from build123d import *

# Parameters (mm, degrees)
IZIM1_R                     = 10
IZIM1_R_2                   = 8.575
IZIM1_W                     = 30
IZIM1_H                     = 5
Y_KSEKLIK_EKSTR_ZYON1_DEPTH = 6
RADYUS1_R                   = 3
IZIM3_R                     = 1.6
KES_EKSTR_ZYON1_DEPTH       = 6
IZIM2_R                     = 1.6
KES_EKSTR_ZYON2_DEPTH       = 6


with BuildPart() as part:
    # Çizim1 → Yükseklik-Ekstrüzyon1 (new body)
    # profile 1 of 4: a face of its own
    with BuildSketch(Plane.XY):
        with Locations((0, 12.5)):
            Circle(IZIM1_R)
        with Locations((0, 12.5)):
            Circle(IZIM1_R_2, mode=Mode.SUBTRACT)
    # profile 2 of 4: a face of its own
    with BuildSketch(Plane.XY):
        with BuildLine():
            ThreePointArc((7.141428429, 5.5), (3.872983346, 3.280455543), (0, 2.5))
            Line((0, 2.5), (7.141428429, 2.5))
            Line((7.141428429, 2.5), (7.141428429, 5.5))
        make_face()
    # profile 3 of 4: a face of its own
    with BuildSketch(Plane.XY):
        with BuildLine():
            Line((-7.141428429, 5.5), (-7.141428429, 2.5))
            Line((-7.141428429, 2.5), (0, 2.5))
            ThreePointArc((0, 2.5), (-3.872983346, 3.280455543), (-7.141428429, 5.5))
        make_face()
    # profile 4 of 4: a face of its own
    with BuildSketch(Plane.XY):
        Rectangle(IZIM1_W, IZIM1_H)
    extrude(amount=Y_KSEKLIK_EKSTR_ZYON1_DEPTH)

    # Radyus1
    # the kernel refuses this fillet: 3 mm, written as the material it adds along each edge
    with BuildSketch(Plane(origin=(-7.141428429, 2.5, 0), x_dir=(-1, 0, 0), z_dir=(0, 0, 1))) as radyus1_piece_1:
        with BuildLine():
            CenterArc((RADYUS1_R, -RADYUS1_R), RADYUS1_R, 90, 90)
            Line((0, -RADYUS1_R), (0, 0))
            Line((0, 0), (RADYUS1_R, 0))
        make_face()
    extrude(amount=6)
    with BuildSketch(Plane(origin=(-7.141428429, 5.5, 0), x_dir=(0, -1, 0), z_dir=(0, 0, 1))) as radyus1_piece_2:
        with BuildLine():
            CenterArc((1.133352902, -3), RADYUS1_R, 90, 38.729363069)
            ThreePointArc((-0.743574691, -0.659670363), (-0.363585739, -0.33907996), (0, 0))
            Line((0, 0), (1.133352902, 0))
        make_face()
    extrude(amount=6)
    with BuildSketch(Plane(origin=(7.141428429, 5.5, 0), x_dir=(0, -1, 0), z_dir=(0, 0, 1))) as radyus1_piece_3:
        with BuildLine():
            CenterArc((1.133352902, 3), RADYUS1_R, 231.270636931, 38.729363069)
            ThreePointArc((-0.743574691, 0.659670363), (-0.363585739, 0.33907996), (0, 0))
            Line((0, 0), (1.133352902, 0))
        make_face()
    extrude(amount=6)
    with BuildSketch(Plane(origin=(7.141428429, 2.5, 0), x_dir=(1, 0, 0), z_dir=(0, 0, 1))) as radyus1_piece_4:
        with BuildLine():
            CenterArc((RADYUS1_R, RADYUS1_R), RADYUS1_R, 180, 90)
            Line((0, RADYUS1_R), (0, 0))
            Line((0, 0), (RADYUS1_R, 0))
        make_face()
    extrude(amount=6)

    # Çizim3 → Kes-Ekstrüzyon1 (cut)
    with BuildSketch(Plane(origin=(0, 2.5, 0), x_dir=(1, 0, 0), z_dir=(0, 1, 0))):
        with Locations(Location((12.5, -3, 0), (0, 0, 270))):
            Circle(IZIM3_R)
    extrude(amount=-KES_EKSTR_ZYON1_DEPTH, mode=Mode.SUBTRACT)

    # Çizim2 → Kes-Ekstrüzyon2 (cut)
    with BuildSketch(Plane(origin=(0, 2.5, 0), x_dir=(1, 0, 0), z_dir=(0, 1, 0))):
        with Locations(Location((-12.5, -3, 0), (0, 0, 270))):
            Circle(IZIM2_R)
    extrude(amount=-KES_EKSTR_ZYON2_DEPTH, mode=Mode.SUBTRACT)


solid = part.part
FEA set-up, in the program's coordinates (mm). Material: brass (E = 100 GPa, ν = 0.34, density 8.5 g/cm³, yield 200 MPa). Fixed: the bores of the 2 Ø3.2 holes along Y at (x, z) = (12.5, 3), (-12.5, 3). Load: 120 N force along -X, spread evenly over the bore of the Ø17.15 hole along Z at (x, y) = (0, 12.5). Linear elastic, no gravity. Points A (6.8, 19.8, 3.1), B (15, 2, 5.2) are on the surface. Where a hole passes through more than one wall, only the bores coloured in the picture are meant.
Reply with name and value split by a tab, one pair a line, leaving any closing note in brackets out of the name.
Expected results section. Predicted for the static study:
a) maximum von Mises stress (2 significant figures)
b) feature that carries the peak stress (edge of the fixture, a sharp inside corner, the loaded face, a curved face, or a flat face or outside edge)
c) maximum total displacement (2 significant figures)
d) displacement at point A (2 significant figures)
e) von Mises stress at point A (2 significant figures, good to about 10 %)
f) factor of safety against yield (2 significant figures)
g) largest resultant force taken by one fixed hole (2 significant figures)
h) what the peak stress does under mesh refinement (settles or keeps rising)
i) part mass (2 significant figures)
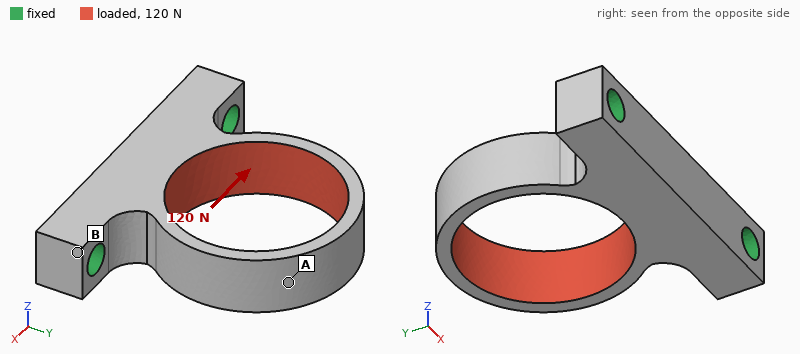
maximum von Mises stress	110 MPa
feature that carries the peak stress	the loaded face
maximum total displacement	76 µm
displacement at point A	74 µm
von Mises stress at point A	45 MPa
factor of safety against yield	1.7
largest resultant force taken by one fixed hole	94 N
what the peak stress does under mesh refinement	settles
part mass	12 g
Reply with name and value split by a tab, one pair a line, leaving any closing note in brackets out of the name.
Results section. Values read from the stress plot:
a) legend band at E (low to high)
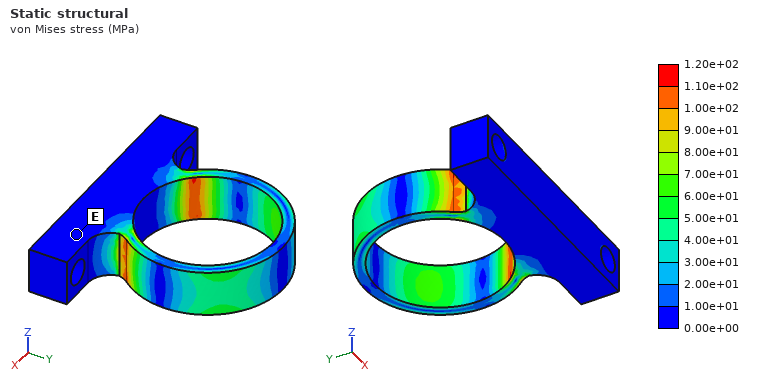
legend band at E	0.00e+00 to 1.00e+01 MPa
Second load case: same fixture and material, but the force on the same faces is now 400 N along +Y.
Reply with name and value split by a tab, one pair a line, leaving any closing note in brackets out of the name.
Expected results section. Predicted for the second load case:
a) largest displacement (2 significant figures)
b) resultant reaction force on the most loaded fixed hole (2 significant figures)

largest displacement	35 µm
resultant reaction force on the most loaded fixed hole	210 N
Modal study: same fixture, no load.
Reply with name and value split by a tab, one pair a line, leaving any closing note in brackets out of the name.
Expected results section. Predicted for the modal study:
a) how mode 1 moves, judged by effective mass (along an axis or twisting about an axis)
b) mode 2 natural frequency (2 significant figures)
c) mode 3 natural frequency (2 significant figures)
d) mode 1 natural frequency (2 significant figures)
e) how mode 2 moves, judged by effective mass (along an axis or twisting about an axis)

how mode 1 moves, judged by effective mass	along X
mode 2 natural frequency	4000 Hz
mode 3 natural frequency	8500 Hz
mode 1 natural frequency	3300 Hz
how mode 2 moves, judged by effective mass	along Z
